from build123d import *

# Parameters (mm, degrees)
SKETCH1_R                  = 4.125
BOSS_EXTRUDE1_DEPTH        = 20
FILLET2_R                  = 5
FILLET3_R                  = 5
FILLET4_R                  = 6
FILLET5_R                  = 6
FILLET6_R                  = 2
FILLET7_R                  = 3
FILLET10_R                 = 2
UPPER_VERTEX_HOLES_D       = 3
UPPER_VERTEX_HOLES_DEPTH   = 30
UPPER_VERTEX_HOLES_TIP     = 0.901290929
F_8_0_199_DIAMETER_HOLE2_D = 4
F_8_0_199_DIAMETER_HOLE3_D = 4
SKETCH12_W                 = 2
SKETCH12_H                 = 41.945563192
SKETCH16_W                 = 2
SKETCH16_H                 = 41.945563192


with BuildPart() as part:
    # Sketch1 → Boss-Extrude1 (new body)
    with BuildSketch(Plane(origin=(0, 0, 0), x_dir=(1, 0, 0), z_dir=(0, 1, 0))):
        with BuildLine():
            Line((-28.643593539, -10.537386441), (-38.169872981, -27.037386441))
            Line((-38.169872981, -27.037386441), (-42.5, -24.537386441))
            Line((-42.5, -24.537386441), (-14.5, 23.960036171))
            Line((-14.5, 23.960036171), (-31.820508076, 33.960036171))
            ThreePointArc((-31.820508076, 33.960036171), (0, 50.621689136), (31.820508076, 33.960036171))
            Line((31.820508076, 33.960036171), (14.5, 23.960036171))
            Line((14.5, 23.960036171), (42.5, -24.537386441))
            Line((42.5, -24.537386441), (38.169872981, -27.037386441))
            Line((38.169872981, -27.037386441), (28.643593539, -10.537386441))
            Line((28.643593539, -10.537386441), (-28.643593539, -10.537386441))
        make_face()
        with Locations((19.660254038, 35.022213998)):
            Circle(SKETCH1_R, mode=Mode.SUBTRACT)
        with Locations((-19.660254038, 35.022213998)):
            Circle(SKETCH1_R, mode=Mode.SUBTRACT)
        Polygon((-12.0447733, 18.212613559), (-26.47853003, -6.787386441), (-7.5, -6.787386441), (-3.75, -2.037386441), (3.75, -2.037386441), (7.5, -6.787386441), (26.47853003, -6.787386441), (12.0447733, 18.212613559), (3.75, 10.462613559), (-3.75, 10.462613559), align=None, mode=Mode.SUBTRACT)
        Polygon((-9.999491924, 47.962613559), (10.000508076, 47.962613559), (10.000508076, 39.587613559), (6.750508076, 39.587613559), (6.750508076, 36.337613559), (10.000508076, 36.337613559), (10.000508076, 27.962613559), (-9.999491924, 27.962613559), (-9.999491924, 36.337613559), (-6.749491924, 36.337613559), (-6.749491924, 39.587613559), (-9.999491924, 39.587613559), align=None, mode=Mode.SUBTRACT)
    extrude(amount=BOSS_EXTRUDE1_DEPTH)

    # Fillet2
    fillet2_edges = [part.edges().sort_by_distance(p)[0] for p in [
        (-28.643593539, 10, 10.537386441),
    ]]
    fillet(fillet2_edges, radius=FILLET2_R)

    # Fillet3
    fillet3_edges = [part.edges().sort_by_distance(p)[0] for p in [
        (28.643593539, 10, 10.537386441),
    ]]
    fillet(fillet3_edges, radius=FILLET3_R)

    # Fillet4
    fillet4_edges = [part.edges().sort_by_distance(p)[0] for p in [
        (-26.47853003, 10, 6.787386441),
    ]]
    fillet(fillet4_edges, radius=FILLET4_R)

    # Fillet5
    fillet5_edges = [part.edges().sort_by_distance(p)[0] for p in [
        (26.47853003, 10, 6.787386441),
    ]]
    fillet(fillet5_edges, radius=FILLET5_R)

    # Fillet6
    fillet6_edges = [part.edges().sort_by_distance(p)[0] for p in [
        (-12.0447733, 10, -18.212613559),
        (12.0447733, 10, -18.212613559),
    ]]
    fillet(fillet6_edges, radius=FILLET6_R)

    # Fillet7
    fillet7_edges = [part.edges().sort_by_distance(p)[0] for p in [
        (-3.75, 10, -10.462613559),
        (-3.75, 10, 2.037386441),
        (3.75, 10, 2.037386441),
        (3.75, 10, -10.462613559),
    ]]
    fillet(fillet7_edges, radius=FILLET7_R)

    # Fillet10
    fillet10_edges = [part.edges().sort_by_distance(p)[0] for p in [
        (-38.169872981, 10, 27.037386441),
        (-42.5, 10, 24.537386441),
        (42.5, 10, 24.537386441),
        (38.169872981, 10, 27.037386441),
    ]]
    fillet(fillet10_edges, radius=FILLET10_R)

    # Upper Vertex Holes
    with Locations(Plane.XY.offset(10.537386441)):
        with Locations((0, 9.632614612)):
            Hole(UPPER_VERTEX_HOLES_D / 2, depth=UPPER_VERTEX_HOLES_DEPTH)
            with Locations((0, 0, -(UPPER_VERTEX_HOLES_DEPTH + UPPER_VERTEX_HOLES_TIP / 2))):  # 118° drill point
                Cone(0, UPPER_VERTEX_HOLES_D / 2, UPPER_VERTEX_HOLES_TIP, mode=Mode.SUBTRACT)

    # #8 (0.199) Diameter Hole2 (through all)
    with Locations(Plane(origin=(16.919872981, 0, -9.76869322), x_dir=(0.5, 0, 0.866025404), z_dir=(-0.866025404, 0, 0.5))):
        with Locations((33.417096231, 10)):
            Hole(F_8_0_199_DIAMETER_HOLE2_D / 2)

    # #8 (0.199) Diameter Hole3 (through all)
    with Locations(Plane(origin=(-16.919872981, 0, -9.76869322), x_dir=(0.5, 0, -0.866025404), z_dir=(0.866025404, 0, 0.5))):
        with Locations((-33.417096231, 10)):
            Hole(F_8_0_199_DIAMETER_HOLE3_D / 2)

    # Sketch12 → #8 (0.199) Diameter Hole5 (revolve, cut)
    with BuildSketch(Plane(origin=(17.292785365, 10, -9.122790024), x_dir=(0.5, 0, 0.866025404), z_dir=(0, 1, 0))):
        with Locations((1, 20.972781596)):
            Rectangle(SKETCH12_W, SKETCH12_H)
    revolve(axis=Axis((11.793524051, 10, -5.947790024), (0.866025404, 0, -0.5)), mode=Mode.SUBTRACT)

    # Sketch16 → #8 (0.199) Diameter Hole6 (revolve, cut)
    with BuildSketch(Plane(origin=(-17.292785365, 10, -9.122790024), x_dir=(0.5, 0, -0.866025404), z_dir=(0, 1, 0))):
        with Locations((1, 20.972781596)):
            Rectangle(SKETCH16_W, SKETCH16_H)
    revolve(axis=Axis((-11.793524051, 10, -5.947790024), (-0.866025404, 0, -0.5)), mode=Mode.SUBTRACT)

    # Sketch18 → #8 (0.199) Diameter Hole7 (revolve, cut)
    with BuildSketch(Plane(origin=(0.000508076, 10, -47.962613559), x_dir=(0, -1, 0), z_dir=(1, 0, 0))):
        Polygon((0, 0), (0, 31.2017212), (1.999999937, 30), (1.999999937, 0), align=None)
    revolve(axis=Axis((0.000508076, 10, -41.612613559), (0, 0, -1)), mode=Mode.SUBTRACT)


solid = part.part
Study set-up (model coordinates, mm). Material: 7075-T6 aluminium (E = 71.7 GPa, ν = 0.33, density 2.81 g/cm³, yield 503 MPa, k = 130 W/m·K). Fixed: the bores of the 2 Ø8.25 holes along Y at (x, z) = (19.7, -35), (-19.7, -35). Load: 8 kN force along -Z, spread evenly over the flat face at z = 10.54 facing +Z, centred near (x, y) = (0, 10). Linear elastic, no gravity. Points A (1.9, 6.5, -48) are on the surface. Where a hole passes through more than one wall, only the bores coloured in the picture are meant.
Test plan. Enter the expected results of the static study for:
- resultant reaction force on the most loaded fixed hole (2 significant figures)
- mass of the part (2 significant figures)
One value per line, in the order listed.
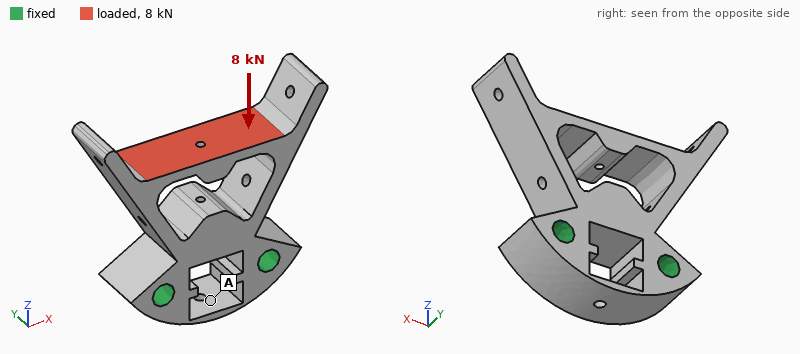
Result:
4.0 kN
100 g
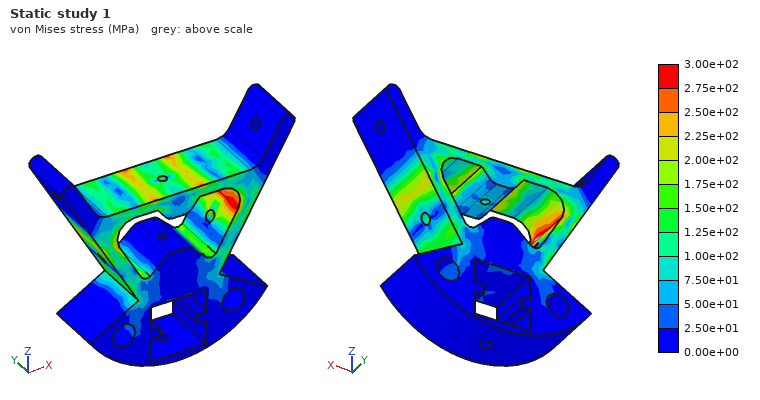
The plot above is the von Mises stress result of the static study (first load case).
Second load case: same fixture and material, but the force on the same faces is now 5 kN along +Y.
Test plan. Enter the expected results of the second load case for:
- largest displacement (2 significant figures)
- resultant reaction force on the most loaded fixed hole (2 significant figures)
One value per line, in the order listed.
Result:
0.56 mm
2.5 kN
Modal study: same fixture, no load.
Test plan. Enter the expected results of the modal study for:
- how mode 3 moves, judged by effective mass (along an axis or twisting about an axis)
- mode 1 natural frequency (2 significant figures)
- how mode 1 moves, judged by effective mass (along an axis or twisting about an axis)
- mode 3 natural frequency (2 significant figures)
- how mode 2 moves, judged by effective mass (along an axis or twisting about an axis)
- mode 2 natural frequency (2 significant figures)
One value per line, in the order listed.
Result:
twisting about Z
1700 Hz
along X
3800 Hz
along Y
3000 Hz
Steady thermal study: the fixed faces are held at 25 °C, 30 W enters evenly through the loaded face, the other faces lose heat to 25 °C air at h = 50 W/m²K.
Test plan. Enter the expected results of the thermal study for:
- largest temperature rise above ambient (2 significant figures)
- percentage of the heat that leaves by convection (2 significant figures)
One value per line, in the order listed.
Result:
43 K
33 %
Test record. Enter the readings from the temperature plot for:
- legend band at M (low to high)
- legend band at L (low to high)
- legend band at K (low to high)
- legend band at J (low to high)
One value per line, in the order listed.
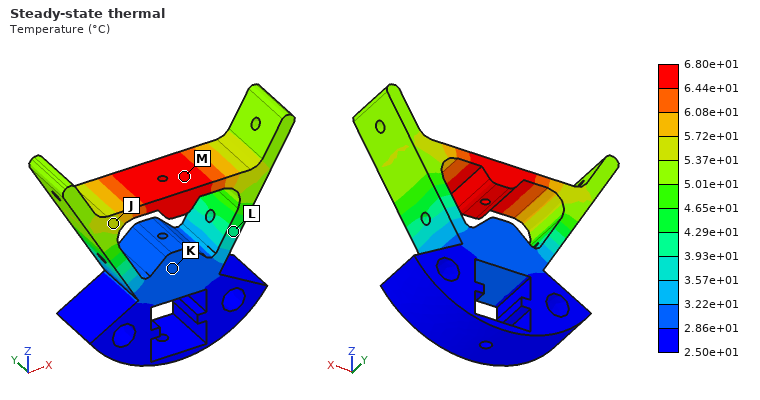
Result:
6.44e+01 to 6.80e+01 °C
3.93e+01 to 4.29e+01 °C
2.86e+01 to 3.22e+01 °C
5.37e+01 to 5.72e+01 °C
